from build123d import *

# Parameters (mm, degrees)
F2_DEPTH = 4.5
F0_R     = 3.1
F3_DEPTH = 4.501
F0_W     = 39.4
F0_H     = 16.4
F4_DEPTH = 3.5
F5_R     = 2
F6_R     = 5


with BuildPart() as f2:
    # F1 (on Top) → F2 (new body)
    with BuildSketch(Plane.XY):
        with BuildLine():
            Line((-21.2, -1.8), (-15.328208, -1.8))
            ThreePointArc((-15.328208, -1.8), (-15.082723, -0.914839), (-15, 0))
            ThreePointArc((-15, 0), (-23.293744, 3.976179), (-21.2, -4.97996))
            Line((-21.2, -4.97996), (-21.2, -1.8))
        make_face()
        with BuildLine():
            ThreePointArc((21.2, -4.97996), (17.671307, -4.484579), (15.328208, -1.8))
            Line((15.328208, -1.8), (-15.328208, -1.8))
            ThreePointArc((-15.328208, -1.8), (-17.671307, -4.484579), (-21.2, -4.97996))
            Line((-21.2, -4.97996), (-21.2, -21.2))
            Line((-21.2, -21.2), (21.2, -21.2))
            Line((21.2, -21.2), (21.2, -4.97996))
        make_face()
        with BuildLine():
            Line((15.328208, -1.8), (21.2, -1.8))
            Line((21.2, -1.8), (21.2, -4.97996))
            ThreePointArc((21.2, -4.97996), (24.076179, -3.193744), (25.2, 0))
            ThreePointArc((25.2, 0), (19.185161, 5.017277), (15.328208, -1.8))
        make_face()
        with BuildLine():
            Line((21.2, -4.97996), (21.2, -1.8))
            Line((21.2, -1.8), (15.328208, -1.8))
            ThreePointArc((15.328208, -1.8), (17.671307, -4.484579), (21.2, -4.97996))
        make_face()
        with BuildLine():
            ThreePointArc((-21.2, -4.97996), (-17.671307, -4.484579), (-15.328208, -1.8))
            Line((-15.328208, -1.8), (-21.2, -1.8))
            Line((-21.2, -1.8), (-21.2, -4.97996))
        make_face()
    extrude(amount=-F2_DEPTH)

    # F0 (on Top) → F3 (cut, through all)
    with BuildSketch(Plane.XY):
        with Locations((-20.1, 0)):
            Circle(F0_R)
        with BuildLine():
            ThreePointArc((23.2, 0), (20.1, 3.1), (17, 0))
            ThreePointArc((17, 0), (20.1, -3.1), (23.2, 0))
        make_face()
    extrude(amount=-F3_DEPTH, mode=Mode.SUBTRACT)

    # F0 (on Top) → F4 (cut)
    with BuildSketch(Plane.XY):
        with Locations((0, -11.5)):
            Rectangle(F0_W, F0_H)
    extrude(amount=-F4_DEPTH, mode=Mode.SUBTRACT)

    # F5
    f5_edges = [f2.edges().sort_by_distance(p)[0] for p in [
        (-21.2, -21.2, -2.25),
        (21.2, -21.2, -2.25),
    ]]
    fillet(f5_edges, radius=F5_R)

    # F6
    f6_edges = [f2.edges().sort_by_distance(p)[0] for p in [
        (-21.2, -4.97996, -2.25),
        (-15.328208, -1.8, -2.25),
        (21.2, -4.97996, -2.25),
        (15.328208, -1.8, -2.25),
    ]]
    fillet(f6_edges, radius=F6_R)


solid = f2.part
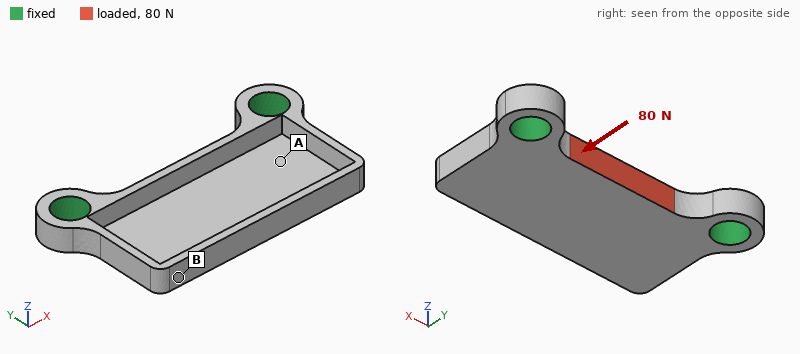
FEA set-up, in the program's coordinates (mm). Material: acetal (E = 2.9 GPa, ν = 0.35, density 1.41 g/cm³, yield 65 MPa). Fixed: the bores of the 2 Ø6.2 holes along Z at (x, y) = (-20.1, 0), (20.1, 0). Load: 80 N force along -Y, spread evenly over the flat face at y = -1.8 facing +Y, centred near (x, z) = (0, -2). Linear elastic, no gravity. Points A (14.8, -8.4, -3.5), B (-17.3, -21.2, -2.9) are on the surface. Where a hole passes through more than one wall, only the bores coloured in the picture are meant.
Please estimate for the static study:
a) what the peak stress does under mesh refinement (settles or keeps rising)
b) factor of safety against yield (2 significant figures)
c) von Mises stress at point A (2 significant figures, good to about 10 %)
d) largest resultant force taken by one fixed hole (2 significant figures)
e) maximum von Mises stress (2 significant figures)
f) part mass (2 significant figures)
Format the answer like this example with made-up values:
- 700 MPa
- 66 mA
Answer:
- settles
- 3.4
- 4.0 MPa
- 47 N
- 19 MPa
- 2.5 g
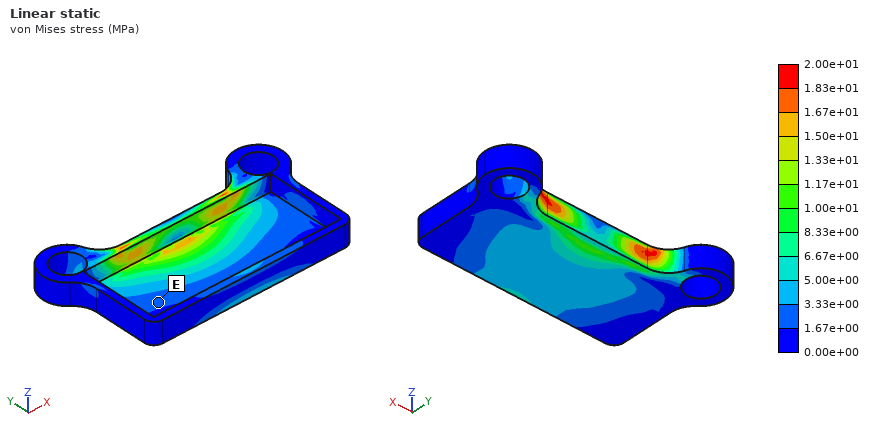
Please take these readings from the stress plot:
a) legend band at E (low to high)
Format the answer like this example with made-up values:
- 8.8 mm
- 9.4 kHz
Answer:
- 1.67e+00 to 3.33e+00 MPa
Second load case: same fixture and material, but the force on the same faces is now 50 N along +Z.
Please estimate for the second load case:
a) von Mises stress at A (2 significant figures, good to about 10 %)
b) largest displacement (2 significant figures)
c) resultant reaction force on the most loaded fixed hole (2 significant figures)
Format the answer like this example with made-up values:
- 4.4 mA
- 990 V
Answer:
- 1.7 MPa
- 0.21 mm
- 25 N
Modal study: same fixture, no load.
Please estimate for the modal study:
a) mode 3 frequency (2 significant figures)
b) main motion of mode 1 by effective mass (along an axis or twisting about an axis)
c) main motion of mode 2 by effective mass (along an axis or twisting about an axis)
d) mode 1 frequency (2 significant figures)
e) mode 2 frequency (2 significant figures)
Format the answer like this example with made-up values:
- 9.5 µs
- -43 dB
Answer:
- 3300 Hz
- along Z
- twisting about Y
- 1300 Hz
- 2400 Hz
